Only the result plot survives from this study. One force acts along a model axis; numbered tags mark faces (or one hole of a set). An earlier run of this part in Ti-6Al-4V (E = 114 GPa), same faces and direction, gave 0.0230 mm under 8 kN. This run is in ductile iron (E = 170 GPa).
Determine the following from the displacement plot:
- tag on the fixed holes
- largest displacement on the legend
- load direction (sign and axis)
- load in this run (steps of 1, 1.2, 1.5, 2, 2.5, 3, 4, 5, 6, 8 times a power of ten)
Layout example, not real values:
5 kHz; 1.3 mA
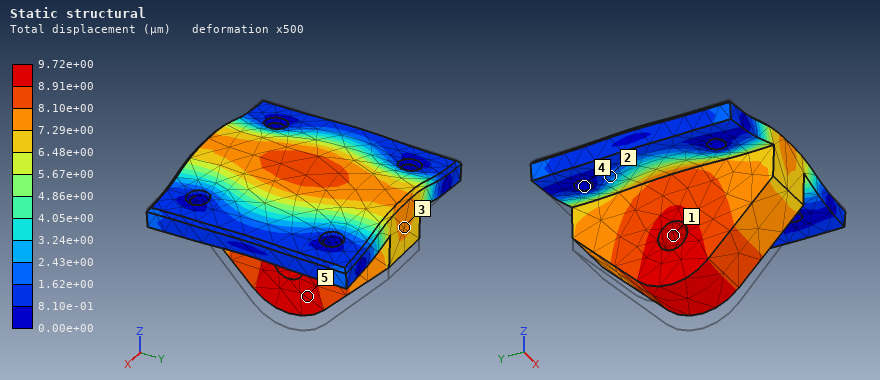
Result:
4; 9.72e+00 µm; +Z; 5 kN
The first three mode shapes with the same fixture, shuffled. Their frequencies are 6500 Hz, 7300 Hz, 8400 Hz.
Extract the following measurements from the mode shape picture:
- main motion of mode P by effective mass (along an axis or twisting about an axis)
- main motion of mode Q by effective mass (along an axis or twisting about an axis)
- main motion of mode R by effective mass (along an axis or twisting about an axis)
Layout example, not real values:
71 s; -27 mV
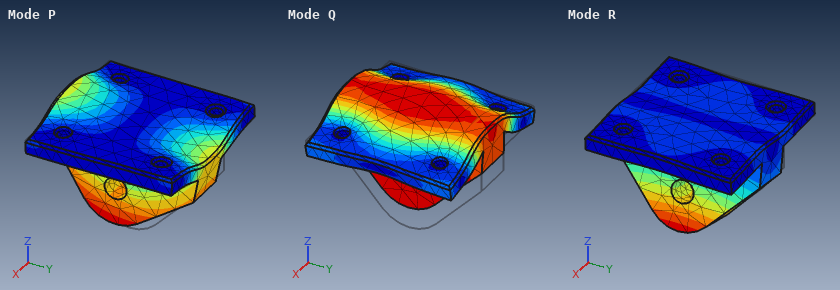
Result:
along Y; along Z; along X
